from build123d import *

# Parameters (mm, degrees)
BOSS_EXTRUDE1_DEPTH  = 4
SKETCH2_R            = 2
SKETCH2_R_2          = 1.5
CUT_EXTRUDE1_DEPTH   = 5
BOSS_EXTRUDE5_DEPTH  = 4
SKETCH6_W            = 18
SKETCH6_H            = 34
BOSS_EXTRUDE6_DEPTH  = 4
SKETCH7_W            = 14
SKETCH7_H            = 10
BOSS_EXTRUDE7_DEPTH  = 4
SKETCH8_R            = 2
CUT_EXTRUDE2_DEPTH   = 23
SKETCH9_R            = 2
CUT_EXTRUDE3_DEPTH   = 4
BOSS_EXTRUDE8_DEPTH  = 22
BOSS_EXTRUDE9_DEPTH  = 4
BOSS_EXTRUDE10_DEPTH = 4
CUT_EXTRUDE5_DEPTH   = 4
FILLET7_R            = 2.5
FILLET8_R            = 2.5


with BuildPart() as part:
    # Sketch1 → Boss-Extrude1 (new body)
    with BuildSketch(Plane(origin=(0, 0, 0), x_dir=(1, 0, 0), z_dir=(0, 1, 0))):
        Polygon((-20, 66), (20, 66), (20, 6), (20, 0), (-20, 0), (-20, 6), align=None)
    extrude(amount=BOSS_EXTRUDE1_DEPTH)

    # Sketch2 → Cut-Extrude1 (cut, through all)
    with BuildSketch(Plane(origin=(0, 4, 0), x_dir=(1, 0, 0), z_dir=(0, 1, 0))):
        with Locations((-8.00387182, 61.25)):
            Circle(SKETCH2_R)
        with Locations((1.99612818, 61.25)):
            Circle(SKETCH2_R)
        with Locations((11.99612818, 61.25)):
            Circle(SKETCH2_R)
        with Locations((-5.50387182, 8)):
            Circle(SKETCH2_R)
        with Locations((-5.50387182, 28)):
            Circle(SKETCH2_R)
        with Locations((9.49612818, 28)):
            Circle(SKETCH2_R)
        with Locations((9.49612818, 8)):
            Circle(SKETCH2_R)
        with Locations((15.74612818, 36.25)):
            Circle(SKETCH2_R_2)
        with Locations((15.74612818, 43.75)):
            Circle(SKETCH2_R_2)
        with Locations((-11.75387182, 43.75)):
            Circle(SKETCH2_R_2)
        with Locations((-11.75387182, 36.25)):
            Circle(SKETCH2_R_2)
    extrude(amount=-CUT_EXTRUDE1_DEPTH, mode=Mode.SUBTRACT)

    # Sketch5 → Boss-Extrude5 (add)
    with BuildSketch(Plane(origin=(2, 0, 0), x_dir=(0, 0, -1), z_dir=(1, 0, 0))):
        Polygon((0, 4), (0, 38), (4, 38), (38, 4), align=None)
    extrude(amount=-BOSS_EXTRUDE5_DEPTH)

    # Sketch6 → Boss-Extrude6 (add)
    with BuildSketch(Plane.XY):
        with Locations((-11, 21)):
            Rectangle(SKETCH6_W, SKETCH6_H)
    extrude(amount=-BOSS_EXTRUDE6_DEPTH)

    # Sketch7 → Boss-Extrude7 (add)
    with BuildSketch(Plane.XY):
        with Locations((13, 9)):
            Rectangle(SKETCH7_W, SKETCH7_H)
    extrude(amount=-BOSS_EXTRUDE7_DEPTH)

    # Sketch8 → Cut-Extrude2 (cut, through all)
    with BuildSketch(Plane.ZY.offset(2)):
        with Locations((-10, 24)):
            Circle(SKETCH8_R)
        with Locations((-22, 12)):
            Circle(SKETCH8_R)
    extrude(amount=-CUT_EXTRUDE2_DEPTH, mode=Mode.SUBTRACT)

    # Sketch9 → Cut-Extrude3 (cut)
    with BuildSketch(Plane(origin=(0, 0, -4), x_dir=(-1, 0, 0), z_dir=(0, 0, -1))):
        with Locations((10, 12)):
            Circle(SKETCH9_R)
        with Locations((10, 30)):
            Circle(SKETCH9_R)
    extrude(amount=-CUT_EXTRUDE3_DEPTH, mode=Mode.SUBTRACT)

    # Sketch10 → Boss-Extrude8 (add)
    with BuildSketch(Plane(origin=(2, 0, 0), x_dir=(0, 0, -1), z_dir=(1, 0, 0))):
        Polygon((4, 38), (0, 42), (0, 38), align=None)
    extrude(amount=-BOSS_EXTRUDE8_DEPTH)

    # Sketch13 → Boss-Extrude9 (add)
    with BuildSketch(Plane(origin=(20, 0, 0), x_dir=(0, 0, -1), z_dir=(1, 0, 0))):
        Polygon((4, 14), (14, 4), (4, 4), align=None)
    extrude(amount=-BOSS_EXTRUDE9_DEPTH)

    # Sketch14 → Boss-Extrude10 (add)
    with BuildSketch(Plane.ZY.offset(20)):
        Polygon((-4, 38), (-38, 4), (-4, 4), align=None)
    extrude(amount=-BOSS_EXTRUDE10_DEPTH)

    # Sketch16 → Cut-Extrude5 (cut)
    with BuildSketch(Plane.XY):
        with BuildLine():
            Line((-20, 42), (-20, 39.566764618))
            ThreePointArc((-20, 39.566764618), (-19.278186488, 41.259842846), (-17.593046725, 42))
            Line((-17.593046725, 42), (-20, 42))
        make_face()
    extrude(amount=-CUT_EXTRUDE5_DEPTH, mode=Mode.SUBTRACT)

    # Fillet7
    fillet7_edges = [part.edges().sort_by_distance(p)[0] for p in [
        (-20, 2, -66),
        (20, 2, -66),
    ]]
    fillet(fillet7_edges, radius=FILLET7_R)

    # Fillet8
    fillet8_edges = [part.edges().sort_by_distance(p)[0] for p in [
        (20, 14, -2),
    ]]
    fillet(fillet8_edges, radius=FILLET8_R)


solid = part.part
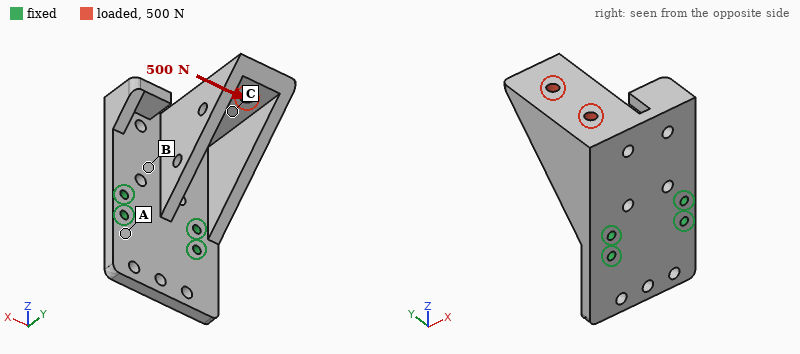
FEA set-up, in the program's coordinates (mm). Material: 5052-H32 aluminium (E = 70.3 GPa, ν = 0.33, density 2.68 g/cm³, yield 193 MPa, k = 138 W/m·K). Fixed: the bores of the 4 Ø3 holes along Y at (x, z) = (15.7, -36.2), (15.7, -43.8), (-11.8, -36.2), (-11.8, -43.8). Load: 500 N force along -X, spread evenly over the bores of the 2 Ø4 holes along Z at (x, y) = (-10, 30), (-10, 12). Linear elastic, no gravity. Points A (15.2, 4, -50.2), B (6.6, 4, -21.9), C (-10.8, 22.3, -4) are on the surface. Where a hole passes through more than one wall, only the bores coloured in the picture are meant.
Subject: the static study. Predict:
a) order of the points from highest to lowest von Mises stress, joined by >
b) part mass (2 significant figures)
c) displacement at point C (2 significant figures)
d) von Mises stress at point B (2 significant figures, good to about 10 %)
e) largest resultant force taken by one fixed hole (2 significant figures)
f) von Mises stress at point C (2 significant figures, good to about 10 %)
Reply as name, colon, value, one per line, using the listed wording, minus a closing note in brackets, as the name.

order of the points from highest to lowest von Mises stress, joined by >: B > C > A
part mass: 49 g
displacement at point C: 0.095 mm
von Mises stress at point B: 32 MPa
largest resultant force taken by one fixed hole: 600 N
von Mises stress at point C: 19 MPa
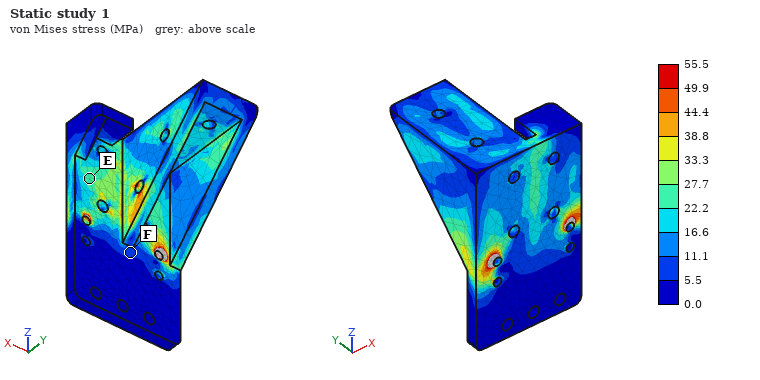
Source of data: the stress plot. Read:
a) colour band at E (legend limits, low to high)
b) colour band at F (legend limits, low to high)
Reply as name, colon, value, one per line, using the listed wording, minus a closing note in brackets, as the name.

colour band at E: 22.2 to 27.7 MPa
colour band at F: 5.5 to 11.1 MPa
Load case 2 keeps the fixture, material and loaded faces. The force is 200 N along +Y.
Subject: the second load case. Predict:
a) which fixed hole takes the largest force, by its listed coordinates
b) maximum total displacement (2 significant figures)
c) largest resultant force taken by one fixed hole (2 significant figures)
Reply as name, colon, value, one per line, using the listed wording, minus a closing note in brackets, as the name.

which fixed hole takes the largest force, by its listed coordinates: (-11.8, -36.2)
maximum total displacement: 0.16 mm
largest resultant force taken by one fixed hole: 460 N
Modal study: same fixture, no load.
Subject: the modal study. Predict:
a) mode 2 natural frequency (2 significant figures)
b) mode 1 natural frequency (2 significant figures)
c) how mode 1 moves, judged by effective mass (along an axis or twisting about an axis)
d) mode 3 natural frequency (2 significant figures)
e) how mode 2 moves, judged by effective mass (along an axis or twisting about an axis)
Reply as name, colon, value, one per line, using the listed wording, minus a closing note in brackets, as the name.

mode 2 natural frequency: 2500 Hz
mode 1 natural frequency: 1500 Hz
how mode 1 moves, judged by effective mass: along Y
mode 3 natural frequency: 6300 Hz
how mode 2 moves, judged by effective mass: along X
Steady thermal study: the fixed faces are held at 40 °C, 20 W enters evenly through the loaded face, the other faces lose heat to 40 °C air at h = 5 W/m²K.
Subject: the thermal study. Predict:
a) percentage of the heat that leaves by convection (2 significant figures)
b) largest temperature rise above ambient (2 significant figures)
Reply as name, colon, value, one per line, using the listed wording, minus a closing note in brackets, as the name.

percentage of the heat that leaves by convection: 3.9 %
largest temperature rise above ambient: 36 K
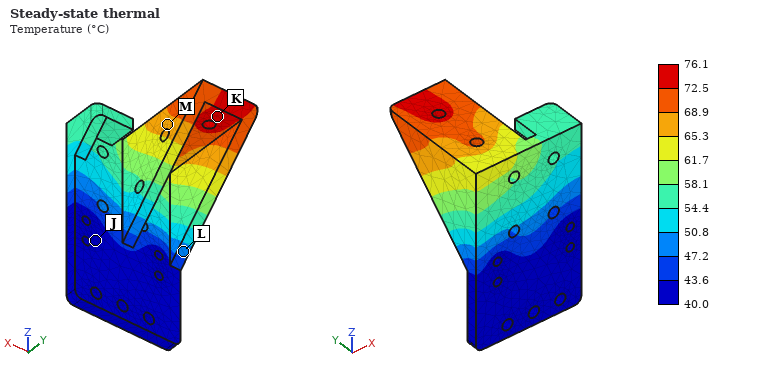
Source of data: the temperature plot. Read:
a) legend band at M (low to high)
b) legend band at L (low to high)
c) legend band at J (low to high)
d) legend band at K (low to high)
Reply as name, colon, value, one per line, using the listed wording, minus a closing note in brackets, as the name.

legend band at M: 65.3 to 68.9 °C
legend band at L: 47.2 to 50.8 °C
legend band at J: 40.0 to 43.6 °C
legend band at K: 72.5 to 76.1 °C
